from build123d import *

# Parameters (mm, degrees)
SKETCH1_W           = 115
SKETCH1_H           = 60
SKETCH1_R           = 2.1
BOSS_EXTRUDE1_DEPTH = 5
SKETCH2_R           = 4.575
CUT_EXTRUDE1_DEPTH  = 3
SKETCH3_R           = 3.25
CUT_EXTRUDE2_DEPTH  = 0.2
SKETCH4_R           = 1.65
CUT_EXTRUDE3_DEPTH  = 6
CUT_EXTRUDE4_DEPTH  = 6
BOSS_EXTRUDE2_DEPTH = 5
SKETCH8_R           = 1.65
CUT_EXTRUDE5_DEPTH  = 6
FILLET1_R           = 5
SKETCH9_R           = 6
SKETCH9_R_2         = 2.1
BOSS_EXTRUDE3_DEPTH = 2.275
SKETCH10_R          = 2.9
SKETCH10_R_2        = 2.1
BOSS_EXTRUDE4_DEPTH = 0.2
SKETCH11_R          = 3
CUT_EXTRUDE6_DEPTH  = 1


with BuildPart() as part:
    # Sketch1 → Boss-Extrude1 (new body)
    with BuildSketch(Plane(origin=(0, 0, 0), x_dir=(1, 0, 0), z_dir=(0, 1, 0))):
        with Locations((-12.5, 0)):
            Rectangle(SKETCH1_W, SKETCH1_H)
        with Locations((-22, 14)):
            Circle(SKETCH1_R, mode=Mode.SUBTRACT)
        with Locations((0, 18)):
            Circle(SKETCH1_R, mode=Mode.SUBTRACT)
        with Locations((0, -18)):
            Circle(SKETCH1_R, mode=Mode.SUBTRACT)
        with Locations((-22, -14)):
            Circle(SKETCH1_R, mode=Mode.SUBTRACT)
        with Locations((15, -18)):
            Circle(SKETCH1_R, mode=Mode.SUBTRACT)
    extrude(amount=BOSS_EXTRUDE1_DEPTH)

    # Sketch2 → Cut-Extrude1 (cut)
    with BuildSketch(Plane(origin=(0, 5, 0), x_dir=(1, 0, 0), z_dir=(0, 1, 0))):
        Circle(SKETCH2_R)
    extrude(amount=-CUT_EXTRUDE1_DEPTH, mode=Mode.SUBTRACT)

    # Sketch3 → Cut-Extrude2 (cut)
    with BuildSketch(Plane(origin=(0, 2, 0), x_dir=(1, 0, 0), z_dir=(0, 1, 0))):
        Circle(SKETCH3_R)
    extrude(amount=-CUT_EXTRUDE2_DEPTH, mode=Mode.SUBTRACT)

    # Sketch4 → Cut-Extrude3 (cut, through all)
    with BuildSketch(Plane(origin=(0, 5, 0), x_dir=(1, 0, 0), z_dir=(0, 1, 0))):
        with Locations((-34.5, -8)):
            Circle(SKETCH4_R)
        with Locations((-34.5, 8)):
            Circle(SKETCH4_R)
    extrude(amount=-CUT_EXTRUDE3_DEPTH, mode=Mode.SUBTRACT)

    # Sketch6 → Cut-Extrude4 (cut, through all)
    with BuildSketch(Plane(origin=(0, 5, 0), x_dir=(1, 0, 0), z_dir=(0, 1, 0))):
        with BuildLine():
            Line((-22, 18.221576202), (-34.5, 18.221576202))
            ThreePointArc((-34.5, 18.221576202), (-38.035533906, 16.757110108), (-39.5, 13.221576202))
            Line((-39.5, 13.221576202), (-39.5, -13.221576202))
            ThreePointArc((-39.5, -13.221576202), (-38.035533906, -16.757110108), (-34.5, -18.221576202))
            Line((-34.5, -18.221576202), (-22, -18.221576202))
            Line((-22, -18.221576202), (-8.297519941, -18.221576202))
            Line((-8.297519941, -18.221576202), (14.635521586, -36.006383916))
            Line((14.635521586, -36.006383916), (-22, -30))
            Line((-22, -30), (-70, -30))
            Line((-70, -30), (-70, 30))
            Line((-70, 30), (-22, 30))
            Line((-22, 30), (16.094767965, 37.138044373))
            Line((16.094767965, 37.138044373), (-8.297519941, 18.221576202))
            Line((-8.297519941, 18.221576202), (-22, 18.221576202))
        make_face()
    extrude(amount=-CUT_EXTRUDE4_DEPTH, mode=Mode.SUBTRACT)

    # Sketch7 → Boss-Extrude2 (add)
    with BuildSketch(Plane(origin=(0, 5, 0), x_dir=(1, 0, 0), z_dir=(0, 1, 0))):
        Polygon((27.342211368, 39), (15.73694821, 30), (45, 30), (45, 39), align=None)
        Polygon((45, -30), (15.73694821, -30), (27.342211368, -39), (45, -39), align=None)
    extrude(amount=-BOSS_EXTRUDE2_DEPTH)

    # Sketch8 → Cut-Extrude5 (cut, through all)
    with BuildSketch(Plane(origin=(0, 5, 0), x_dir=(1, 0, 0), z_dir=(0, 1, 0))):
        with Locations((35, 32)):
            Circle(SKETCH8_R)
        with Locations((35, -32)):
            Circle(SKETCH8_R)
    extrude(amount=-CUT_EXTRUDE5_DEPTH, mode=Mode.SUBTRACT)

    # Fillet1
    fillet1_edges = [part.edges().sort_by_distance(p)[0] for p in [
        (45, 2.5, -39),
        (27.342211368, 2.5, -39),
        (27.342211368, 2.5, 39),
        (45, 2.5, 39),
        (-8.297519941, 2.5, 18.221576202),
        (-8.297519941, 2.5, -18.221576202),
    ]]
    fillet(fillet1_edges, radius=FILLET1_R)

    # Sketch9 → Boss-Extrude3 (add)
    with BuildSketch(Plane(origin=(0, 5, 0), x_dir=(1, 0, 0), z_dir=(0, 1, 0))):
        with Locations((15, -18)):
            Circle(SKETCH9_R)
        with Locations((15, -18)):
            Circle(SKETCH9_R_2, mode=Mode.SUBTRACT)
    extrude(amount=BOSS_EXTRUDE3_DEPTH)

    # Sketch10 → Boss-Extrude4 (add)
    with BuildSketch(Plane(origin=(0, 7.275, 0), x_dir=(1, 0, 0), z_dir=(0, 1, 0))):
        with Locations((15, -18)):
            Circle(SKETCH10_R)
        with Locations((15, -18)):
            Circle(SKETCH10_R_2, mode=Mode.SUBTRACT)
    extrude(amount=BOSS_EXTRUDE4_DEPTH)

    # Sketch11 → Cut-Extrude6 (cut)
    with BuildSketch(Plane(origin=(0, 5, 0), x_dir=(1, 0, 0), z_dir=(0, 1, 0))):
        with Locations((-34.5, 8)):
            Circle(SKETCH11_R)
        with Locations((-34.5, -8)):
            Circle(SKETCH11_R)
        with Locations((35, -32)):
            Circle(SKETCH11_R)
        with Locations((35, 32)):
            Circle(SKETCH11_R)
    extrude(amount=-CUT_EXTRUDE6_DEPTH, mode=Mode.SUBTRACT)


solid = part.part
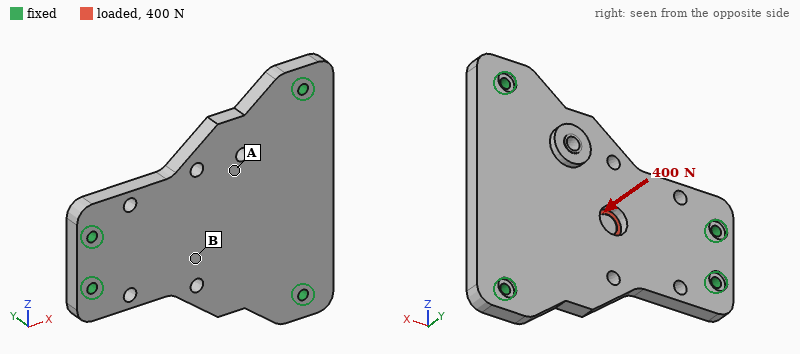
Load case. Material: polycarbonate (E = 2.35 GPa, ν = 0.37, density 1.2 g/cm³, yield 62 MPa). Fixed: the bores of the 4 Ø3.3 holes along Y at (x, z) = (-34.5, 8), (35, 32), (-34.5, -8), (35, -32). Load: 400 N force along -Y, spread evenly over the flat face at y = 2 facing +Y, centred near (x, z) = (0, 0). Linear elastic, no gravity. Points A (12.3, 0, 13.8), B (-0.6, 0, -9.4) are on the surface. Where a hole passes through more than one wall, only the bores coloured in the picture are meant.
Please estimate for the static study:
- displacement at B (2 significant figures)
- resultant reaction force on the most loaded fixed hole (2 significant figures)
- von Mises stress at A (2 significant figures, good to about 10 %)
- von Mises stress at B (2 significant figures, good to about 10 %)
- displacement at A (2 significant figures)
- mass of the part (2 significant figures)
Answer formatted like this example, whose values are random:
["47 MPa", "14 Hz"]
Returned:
["1.1 mm", "110 N", "6.0 MPa", "20 MPa", "0.82 mm", "27 g"]
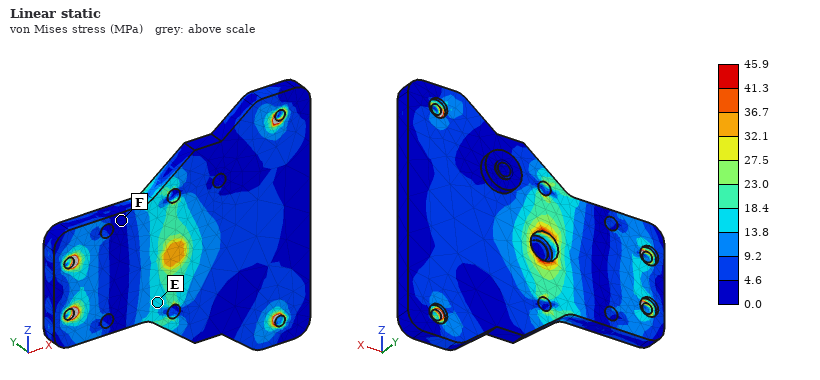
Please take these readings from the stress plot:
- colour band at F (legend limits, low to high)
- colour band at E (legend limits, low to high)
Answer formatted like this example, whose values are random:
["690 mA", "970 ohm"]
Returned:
["0.0 to 4.6 MPa", "13.8 to 18.4 MPa"]
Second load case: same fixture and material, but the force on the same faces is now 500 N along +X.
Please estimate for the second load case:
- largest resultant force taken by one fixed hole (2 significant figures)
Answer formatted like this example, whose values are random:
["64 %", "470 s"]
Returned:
["150 N"]
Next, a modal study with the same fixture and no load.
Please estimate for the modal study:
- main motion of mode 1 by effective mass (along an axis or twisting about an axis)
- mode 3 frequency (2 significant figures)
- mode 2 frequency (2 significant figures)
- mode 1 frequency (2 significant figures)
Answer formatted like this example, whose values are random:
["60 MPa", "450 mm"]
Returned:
["along Y", "1700 Hz", "1700 Hz", "1000 Hz"]
